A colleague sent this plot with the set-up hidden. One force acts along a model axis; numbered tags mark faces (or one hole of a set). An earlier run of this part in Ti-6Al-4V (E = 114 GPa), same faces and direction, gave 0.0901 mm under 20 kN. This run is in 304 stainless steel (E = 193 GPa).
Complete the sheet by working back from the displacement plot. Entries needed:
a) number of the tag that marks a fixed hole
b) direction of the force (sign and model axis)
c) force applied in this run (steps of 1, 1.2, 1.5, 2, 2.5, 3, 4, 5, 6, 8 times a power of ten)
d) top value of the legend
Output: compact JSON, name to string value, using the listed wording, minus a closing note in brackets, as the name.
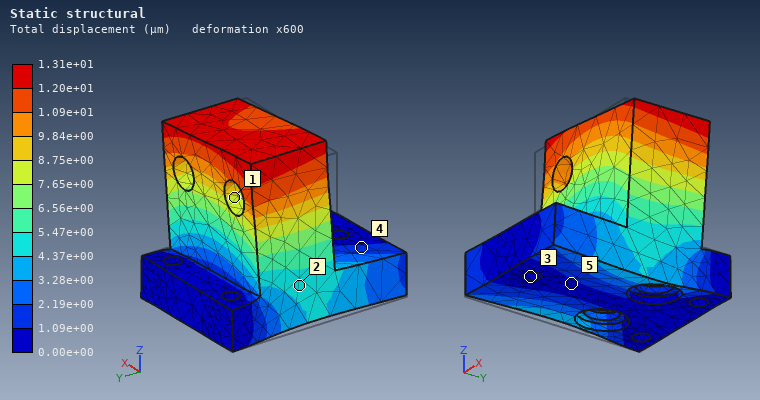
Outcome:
{"number of the tag that marks a fixed hole": "3", "direction of the force": "+X", "force applied in this run": "5 kN", "top value of the legend": "1.31e+01 µm"}
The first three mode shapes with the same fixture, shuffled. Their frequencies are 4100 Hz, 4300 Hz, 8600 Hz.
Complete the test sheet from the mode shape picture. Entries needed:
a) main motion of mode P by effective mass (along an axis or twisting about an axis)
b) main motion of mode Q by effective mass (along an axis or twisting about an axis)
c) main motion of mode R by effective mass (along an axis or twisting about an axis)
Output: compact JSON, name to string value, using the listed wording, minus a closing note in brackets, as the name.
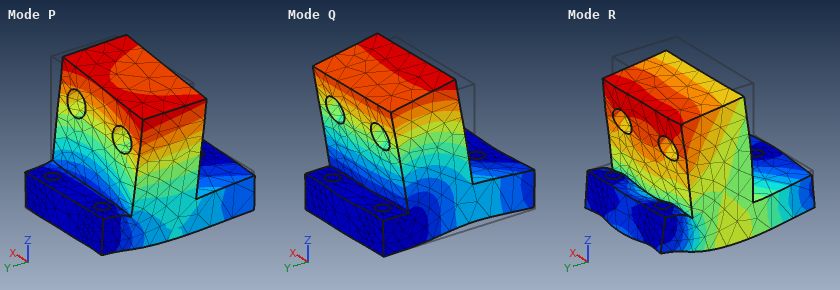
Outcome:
{"main motion of mode P by effective mass": "along X", "main motion of mode Q by effective mass": "along Y", "main motion of mode R by effective mass": "along Z"}
